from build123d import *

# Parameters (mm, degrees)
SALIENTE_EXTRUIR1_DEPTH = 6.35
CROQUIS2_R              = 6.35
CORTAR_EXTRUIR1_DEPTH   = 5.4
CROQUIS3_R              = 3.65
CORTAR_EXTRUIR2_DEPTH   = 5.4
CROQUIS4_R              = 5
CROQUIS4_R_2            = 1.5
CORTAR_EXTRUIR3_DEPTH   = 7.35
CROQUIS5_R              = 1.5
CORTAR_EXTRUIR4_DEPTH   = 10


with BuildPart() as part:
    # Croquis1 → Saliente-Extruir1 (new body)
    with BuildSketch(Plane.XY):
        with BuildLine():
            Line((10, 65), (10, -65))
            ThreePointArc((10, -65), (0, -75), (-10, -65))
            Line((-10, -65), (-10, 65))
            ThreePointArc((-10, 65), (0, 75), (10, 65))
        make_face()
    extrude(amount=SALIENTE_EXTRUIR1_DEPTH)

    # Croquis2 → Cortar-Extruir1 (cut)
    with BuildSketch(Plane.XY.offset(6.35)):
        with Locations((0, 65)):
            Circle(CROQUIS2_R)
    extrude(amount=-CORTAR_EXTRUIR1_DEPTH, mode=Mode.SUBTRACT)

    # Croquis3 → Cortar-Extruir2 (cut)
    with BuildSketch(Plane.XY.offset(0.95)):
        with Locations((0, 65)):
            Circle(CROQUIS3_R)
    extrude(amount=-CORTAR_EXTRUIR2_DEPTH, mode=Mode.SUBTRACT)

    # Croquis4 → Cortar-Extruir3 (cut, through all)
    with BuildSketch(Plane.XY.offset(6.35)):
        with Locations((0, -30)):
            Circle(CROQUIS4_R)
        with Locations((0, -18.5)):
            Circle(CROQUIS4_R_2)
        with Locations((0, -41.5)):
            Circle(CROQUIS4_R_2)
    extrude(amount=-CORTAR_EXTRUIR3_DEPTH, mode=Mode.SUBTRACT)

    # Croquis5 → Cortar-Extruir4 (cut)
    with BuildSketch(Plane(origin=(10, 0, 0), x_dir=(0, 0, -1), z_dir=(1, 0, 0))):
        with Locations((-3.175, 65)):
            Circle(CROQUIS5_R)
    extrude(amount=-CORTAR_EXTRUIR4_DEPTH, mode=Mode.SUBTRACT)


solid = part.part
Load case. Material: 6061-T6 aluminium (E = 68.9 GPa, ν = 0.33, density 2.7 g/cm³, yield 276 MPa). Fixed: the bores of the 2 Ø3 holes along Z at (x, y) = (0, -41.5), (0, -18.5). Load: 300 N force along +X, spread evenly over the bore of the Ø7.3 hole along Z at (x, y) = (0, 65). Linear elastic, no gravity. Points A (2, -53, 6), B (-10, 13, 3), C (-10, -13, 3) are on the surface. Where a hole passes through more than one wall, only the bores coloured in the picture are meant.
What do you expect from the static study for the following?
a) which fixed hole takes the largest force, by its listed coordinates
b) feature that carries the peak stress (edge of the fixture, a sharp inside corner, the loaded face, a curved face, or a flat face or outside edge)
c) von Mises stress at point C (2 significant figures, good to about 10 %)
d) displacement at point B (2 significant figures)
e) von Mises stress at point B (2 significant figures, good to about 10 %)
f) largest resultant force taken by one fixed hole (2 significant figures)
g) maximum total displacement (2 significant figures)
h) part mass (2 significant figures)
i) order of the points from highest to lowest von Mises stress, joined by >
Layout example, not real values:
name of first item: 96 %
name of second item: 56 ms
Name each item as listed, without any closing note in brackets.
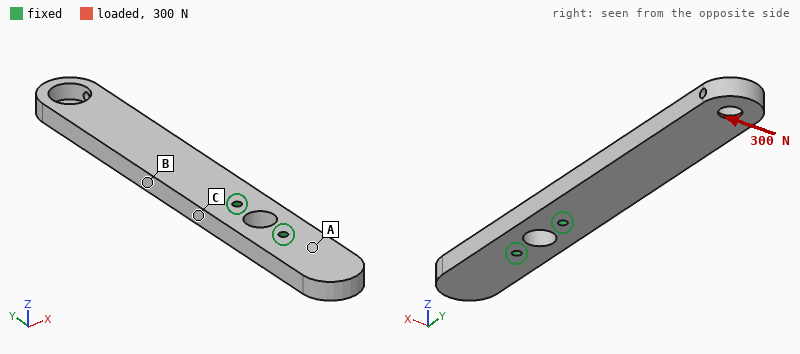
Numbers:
which fixed hole takes the largest force, by its listed coordinates: (0, -18.5)
feature that carries the peak stress: edge of the fixture
von Mises stress at point C: 57 MPa
displacement at point B: 0.087 mm
von Mises stress at point B: 37 MPa
largest resultant force taken by one fixed hole: 1.0 kN
maximum total displacement: 0.37 mm
part mass: 46 g
order of the points from highest to lowest von Mises stress, joined by >: C > B > A
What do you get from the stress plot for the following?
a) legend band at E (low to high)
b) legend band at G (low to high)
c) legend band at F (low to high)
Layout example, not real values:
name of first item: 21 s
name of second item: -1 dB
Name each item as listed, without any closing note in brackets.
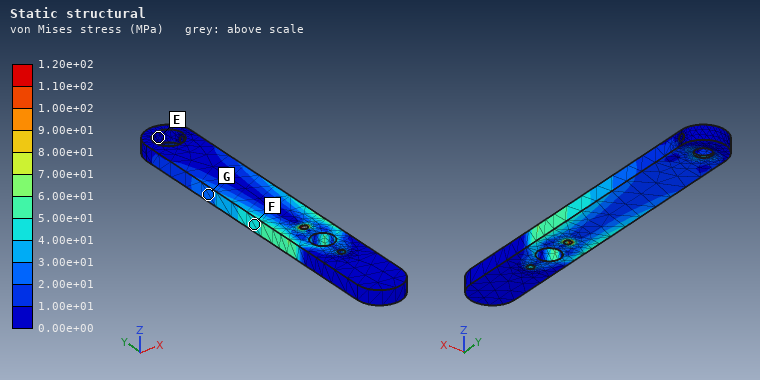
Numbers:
legend band at E: 0.00e+00 to 1.00e+01 MPa
legend band at G: 2.00e+01 to 3.00e+01 MPa
legend band at F: 4.00e+01 to 5.00e+01 MPa
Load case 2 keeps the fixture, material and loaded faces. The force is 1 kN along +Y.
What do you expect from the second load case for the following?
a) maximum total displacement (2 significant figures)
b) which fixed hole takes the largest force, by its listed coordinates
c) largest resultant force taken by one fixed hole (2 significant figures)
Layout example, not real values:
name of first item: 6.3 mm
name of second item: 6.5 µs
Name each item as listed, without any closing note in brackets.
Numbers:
maximum total displacement: 0.41 mm
which fixed hole takes the largest force, by its listed coordinates: (0, -18.5)
largest resultant force taken by one fixed hole: 850 N
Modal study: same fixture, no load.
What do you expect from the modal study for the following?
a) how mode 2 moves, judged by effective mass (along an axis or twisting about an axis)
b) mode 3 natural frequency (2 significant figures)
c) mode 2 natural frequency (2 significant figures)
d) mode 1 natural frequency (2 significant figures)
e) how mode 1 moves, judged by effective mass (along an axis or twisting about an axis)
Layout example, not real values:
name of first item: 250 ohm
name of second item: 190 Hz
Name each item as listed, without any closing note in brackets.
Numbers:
how mode 2 moves, judged by effective mass: along X
mode 3 natural frequency: 3900 Hz
mode 2 natural frequency: 1600 Hz
mode 1 natural frequency: 670 Hz
how mode 1 moves, judged by effective mass: along Z
